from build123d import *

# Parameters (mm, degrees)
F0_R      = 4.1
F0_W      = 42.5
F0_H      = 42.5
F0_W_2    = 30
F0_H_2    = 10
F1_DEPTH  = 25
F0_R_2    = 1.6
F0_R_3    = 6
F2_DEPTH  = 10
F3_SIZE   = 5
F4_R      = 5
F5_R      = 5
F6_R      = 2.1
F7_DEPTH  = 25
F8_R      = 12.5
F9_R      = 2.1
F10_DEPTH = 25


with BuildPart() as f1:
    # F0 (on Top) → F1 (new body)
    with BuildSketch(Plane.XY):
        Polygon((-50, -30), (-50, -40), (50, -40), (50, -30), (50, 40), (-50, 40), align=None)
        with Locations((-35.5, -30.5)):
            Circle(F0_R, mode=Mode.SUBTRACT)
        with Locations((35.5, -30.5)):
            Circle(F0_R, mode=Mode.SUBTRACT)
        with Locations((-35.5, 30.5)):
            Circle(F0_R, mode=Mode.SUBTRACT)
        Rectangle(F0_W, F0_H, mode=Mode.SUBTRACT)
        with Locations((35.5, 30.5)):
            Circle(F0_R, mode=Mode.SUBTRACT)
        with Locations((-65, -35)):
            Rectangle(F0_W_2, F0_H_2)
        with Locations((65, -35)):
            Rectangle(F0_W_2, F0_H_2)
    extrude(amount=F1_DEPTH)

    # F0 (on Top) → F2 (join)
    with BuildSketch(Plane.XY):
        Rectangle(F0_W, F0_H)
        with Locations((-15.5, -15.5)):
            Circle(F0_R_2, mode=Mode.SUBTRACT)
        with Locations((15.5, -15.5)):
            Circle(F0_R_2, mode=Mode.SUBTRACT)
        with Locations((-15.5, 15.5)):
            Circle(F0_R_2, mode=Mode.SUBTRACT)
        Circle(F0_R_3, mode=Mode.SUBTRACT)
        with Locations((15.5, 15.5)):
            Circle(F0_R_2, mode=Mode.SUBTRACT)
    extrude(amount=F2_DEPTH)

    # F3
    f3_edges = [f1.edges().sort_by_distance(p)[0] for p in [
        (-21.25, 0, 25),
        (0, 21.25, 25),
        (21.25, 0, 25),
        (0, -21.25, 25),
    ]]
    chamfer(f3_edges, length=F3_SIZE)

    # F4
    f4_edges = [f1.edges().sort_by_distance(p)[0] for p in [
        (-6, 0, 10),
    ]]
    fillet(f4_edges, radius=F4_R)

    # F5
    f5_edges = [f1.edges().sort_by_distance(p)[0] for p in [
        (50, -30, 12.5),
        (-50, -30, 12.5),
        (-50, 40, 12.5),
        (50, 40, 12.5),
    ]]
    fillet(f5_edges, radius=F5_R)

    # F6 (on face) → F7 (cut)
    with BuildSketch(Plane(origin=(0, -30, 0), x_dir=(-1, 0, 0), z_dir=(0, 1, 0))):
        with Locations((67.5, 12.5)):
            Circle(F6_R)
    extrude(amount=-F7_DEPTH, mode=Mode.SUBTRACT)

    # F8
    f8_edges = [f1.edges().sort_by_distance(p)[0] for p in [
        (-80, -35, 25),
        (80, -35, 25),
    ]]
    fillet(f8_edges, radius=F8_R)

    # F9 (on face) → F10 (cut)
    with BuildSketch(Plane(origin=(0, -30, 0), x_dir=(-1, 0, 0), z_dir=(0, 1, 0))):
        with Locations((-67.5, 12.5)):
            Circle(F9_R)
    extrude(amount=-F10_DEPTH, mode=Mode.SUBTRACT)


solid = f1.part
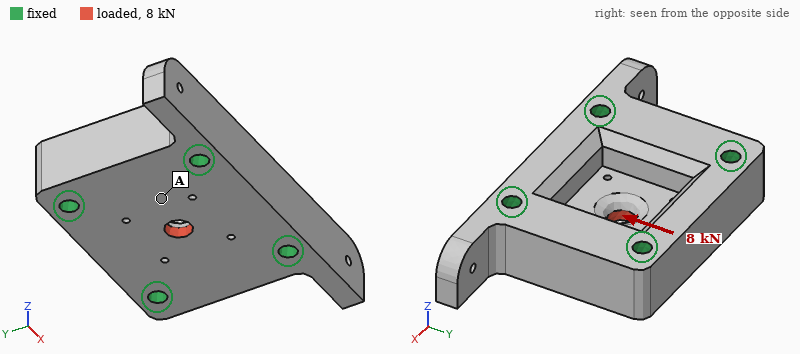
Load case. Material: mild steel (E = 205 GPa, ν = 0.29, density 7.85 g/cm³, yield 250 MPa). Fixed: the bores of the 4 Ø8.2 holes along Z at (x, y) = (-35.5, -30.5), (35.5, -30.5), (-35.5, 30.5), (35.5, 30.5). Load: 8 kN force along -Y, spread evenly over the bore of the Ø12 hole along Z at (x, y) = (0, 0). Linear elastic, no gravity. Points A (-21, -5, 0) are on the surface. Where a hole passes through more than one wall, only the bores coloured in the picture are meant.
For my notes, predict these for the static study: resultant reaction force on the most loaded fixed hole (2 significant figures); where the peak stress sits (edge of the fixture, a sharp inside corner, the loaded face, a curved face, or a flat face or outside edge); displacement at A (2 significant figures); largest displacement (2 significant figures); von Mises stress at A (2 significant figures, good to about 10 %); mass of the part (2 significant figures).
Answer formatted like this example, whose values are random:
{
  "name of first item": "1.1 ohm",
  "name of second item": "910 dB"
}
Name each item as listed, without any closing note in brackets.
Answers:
{
  "resultant reaction force on the most loaded fixed hole": "2.4 kN",
  "where the peak stress sits": "the loaded face",
  "displacement at A": "0.76 µm",
  "largest displacement": "3.5 µm",
  "von Mises stress at A": "6.8 MPa",
  "mass of the part": "1.4 kg"
}
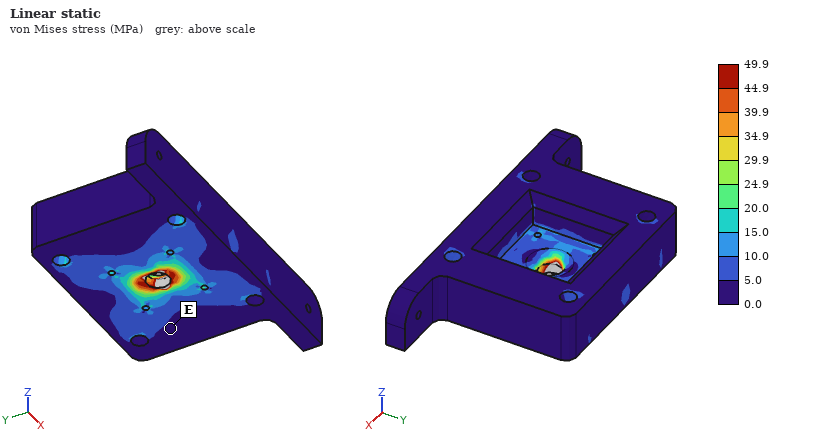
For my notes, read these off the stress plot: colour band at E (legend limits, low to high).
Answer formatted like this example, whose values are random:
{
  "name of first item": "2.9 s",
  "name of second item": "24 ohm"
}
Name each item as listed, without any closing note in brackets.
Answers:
{
  "colour band at E": "0.0 to 5.0 MPa"
}
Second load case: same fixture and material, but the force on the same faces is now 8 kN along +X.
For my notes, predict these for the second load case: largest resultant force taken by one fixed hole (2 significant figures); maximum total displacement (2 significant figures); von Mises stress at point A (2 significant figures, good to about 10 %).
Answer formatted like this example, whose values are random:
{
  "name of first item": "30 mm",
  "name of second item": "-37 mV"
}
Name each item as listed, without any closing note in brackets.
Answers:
{
  "largest resultant force taken by one fixed hole": "2.2 kN",
  "maximum total displacement": "3.2 µm",
  "von Mises stress at point A": "8.0 MPa"
}
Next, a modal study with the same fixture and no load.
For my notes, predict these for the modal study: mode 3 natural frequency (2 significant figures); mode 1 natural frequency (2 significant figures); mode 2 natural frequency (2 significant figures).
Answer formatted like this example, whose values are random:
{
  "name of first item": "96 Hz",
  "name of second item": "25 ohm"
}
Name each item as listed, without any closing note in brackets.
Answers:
{
  "mode 3 natural frequency": "11 kHz",
  "mode 1 natural frequency": "7300 Hz",
  "mode 2 natural frequency": "7300 Hz"
}
